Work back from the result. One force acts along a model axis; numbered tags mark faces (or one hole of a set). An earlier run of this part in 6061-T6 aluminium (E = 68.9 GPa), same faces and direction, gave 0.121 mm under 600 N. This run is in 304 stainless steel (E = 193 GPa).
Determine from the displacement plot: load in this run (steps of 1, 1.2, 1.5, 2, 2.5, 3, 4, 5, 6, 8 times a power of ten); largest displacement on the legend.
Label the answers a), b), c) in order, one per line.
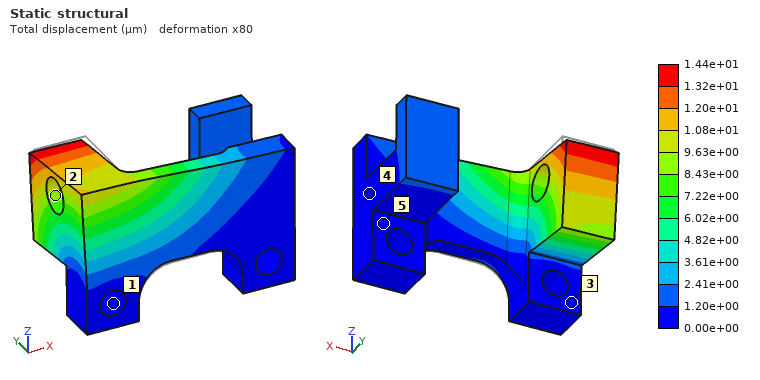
a) 200 N
b) 1.44e+01 µm
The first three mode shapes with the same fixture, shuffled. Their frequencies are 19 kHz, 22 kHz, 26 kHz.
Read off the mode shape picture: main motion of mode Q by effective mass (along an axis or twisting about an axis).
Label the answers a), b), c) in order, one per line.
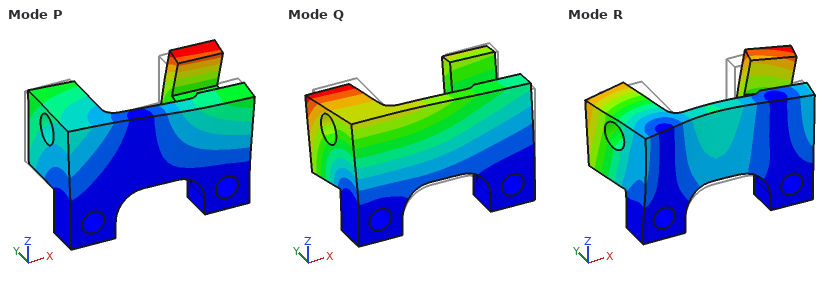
a) along Y
